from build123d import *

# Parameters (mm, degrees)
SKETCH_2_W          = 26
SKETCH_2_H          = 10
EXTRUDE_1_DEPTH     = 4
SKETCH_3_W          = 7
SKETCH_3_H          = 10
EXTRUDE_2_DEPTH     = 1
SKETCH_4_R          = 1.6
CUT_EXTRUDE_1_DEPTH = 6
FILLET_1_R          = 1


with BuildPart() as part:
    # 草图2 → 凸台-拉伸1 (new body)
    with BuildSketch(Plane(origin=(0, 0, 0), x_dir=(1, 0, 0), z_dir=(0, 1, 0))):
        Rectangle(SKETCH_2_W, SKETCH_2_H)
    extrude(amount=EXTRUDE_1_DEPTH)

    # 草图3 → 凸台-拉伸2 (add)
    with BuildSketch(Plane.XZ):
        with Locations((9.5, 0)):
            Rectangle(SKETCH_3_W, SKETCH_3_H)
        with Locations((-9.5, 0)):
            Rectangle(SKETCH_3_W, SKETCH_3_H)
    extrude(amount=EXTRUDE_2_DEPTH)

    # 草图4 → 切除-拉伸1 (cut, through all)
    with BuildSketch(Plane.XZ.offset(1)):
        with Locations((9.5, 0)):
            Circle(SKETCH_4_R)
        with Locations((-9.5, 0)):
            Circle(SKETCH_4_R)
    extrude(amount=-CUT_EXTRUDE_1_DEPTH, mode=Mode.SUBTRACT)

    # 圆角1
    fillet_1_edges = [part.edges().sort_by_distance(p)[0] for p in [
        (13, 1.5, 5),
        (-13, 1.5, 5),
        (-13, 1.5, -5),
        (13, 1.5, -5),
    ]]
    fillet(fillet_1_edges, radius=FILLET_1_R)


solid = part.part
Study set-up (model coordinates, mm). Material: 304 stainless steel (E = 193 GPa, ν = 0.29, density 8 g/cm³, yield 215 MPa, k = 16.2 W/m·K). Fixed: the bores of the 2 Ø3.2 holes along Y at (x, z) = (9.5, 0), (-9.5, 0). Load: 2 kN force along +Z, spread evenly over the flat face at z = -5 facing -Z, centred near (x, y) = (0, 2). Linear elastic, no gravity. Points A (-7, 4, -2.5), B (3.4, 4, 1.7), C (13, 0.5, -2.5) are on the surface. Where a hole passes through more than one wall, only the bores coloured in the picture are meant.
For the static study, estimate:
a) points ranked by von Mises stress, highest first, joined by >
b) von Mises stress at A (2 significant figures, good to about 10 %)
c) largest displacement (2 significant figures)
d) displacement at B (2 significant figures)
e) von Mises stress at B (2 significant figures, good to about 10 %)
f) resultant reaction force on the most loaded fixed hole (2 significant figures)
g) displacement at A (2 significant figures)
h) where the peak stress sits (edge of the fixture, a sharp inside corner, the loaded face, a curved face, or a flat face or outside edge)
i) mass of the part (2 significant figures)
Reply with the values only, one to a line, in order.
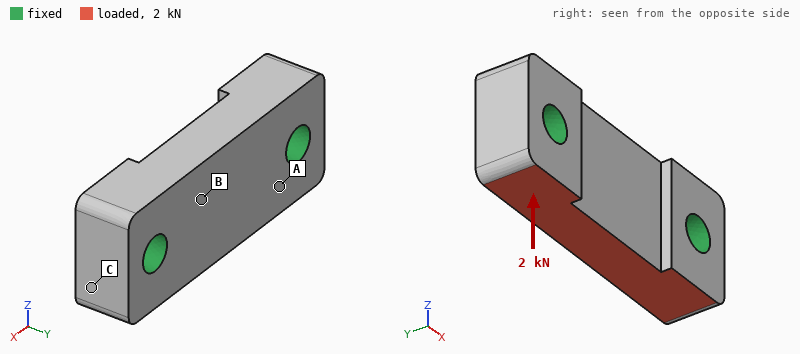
A > B > C
31 MPa
2.0 µm
1.4 µm
17 MPa
1.0 kN
0.73 µm
edge of the fixture
8.8 g
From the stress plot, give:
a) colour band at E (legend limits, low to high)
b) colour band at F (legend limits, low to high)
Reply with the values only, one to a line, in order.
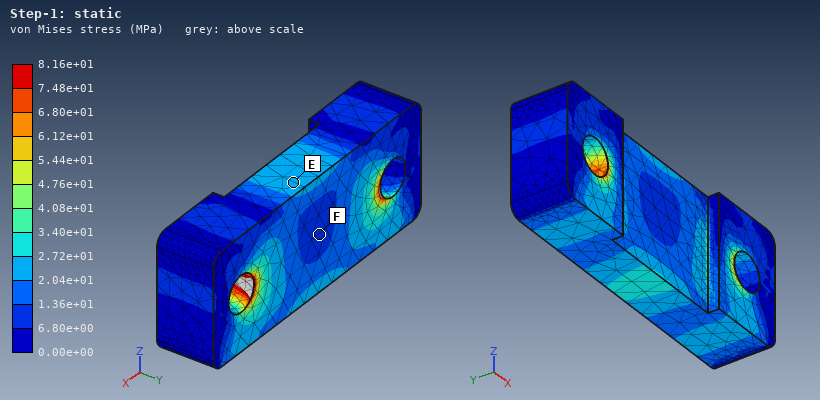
2.04e+01 to 2.72e+01 MPa
6.80e+00 to 1.36e+01 MPa
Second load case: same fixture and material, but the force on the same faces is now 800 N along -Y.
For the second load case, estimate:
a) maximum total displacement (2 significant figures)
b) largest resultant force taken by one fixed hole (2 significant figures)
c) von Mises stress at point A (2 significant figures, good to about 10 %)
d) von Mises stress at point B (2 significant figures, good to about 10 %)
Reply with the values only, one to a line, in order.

3.7 µm
400 N
35 MPa
16 MPa
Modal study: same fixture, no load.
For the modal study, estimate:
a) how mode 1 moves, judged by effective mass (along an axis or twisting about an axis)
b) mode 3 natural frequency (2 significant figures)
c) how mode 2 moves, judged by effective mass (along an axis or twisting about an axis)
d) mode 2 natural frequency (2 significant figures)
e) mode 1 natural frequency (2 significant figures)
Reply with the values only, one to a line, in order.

along Y
66 kHz
along Z
62 kHz
54 kHz
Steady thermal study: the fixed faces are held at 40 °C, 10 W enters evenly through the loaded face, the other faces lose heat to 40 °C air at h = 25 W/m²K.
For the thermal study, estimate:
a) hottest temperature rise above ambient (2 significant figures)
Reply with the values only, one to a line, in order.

43 K
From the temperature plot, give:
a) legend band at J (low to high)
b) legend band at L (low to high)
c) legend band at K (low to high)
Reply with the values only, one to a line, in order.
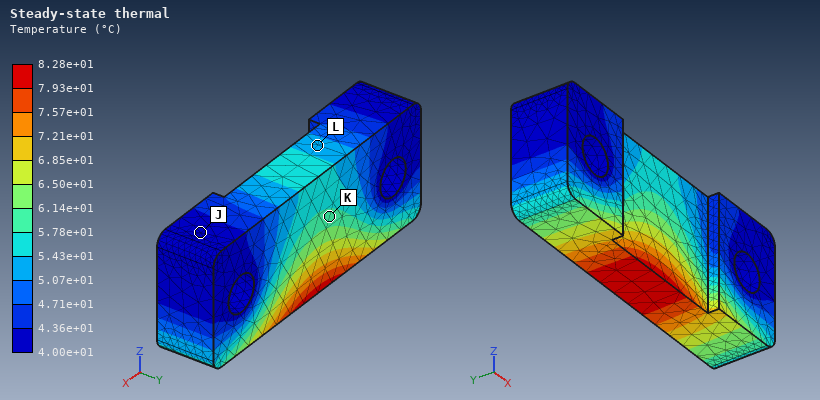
4.00e+01 to 4.36e+01 °C
5.07e+01 to 5.43e+01 °C
5.78e+01 to 6.14e+01 °C
